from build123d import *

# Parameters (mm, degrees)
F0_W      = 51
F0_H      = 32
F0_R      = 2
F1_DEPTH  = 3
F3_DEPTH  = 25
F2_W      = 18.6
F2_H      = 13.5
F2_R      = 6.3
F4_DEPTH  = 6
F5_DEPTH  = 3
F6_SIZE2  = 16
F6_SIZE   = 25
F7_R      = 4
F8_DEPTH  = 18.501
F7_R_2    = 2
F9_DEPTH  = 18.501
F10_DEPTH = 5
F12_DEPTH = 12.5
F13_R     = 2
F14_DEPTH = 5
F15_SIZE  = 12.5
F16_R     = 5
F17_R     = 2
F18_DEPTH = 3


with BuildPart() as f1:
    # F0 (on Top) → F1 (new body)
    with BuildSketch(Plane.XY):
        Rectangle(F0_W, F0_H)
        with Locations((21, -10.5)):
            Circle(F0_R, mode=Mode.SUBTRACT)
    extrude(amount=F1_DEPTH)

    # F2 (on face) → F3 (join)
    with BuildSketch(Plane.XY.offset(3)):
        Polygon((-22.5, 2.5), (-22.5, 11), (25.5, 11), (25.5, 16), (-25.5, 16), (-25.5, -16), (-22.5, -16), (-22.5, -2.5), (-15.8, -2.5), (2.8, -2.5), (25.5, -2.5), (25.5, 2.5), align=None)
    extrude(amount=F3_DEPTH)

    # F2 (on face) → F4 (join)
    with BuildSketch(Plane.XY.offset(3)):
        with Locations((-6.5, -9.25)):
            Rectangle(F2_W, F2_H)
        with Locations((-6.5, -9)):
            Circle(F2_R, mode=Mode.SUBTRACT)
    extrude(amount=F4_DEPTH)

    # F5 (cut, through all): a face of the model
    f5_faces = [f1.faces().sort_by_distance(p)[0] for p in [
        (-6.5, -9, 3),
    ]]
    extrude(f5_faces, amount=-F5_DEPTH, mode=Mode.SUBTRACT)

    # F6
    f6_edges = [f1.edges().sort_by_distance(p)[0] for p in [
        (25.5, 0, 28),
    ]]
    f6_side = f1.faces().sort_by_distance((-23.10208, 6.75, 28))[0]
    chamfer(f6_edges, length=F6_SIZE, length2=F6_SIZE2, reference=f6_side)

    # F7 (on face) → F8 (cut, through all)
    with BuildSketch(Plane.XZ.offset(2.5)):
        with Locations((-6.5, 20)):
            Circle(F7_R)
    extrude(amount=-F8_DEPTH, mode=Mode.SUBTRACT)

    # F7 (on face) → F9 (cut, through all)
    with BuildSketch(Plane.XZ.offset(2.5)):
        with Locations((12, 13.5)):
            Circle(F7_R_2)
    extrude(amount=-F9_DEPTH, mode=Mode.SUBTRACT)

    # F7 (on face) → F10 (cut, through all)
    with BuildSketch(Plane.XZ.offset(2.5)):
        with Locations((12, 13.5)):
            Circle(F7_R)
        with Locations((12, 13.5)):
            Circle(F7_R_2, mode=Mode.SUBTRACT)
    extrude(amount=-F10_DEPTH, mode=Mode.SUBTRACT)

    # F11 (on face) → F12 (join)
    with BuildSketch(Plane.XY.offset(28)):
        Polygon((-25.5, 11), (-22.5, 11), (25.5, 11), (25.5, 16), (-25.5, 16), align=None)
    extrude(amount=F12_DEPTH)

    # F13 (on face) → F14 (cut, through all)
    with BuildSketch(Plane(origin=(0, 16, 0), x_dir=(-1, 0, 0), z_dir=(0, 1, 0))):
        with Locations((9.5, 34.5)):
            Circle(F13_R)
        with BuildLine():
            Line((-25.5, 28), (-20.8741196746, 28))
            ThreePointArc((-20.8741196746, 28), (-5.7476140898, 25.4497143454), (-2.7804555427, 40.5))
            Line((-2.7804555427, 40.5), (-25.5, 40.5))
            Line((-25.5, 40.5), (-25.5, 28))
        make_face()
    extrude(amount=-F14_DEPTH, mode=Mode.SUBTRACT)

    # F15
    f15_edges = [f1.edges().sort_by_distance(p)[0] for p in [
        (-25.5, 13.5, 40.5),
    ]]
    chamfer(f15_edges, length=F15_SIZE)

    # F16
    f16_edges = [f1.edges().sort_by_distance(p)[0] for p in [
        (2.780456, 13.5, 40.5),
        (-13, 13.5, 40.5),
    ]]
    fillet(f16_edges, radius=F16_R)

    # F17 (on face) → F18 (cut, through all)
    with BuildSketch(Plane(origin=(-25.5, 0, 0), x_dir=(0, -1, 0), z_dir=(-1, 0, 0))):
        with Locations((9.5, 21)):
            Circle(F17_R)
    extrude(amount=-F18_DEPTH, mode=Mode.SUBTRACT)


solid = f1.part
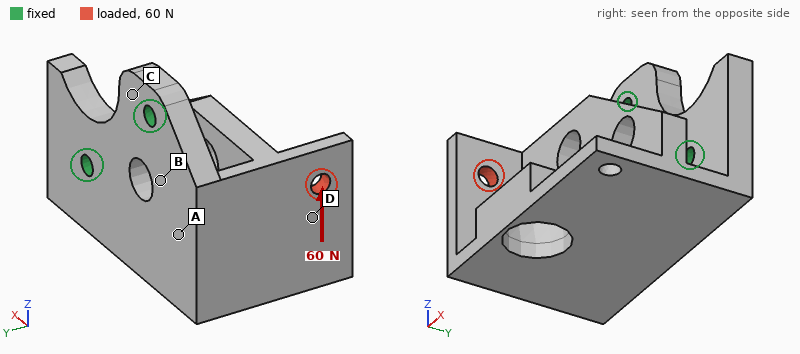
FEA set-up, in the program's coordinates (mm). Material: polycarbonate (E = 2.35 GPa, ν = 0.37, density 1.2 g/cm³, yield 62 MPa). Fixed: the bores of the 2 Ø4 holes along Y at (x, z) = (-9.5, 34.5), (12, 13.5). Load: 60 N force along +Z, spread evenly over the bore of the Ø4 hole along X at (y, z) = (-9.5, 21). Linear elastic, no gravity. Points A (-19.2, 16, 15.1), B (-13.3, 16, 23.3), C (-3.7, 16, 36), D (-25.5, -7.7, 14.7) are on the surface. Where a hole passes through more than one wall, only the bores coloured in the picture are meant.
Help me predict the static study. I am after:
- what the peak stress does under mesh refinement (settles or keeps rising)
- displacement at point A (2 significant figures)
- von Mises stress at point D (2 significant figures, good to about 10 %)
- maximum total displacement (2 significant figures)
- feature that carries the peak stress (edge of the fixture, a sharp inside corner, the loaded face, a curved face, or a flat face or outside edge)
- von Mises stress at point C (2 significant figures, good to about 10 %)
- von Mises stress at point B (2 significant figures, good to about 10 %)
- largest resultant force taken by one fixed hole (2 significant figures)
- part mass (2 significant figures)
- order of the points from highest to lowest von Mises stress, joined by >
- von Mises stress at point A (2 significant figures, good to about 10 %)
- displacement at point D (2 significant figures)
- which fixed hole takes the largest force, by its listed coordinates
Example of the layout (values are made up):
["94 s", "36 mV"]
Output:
["keeps rising", "0.16 mm", "1.9 MPa", "0.73 mm", "edge of the fixture", "0.80 MPa", "4.3 MPa", "76 N", "22 g", "B > A > D > C", "2.7 MPa", "0.48 mm", "(-9.5, 34.5)"]
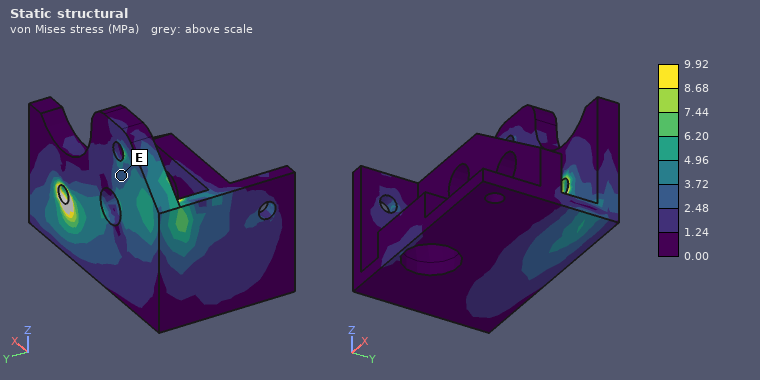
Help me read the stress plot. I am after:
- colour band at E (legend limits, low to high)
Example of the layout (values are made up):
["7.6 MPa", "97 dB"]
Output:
["2.48 to 3.72 MPa"]
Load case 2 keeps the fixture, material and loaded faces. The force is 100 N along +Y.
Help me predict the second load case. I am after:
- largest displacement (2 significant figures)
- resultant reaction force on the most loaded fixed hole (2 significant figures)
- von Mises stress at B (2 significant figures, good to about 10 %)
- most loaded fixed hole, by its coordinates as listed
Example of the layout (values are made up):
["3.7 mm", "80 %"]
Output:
["0.63 mm", "88 N", "4.4 MPa", "(-9.5, 34.5)"]
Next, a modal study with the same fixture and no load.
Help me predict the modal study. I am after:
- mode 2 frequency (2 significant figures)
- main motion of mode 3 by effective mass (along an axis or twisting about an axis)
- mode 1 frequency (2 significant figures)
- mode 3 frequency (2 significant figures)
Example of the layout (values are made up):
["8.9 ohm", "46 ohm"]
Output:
["980 Hz", "along Y", "520 Hz", "1500 Hz"]
